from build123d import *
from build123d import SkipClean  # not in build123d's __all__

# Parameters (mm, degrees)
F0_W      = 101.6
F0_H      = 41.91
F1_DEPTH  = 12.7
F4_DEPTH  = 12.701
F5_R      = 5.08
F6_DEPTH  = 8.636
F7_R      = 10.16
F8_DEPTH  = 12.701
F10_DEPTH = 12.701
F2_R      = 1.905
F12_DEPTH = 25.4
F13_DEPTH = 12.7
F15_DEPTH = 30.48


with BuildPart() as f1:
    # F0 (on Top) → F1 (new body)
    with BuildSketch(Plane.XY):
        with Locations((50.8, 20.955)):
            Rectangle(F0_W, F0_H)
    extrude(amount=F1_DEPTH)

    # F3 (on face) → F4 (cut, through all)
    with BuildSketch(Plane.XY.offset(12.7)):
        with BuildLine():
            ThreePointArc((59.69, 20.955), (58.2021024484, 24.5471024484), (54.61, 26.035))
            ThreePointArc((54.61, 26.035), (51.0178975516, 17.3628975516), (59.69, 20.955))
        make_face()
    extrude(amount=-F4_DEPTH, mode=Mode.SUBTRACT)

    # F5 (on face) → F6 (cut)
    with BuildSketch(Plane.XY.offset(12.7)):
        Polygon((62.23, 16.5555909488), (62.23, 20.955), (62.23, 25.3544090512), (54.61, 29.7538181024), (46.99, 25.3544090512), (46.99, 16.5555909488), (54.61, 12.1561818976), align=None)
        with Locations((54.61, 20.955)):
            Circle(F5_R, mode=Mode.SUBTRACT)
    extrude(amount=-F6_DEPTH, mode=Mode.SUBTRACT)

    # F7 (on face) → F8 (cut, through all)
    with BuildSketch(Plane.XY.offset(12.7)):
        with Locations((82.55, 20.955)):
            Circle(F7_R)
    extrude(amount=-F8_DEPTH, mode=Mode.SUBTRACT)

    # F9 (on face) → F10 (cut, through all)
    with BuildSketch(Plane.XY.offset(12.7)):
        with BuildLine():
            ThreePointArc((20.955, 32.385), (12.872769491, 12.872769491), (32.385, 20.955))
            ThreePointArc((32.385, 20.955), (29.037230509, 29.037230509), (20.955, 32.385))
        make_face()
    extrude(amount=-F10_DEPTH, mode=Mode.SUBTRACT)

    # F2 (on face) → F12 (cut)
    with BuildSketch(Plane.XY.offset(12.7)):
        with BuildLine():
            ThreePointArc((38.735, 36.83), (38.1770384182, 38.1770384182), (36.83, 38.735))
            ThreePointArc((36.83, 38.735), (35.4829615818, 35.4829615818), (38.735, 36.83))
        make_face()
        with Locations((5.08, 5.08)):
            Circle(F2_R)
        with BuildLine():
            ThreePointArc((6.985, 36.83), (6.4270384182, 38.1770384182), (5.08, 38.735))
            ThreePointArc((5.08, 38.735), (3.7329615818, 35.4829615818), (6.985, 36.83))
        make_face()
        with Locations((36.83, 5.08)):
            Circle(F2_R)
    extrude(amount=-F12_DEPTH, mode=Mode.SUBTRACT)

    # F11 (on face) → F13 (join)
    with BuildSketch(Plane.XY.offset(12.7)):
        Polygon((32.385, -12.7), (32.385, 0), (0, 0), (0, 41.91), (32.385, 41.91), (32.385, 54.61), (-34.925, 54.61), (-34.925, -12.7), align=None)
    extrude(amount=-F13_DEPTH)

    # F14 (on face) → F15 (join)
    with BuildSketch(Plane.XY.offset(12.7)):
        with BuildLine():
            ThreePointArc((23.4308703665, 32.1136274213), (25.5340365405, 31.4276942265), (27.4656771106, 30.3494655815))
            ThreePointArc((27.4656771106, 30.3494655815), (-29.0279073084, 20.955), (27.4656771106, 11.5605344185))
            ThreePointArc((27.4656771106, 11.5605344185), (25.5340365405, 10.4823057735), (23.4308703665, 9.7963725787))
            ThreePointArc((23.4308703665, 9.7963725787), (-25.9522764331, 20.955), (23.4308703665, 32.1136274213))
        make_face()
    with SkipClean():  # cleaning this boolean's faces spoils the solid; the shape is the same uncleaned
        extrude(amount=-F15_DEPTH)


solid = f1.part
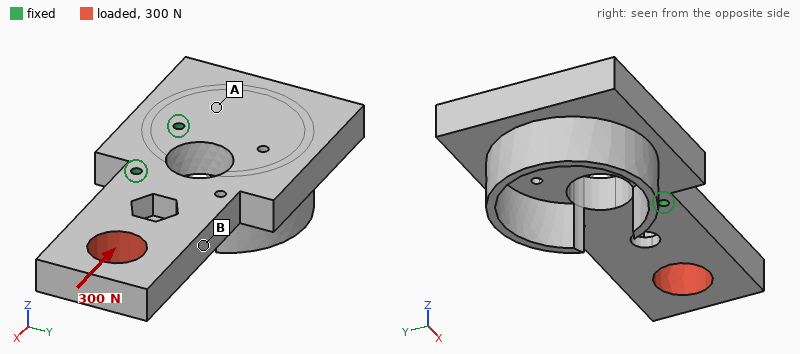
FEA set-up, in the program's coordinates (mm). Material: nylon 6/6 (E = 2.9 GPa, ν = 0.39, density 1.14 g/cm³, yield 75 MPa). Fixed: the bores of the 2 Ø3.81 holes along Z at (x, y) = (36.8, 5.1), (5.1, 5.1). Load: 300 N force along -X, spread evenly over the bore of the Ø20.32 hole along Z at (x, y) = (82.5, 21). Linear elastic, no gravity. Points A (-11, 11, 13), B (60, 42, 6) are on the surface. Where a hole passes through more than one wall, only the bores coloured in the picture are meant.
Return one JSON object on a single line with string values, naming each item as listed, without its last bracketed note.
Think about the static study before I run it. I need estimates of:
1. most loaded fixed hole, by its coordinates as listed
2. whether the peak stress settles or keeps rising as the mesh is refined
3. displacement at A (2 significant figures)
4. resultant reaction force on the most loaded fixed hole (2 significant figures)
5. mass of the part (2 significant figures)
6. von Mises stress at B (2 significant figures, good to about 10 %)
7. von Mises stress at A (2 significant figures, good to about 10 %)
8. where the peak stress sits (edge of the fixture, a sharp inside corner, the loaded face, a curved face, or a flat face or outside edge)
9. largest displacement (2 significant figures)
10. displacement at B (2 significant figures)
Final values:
{"most loaded fixed hole, by its coordinates as listed": "(36.8, 5.1)", "whether the peak stress settles or keeps rising as the mesh is refined": "keeps rising", "displacement at A": "14 µm", "resultant reaction force on the most loaded fixed hole": "220 N", "mass of the part": "100 g", "von Mises stress at B": "0.79 MPa", "von Mises stress at A": "0.32 MPa", "where the peak stress sits": "edge of the fixture", "largest displacement": "86 µm", "displacement at B": "55 µm"}
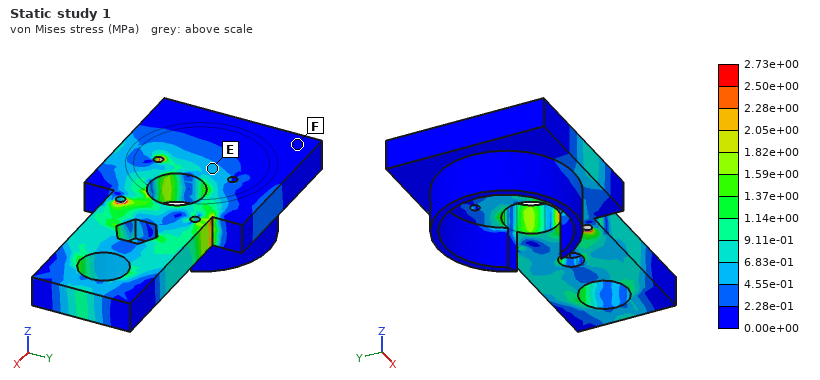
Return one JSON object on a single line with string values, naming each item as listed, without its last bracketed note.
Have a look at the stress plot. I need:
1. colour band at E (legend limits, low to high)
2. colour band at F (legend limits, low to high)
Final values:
{"colour band at E": "4.55e-01 to 6.83e-01 MPa", "colour band at F": "0.00e+00 to 2.28e-01 MPa"}
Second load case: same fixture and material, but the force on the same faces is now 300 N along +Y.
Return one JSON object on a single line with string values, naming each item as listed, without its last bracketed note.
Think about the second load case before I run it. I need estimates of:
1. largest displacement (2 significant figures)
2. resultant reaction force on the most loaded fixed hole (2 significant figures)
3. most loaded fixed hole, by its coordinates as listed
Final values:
{"largest displacement": "0.39 mm", "resultant reaction force on the most loaded fixed hole": "720 N", "most loaded fixed hole, by its coordinates as listed": "(36.8, 5.1)"}
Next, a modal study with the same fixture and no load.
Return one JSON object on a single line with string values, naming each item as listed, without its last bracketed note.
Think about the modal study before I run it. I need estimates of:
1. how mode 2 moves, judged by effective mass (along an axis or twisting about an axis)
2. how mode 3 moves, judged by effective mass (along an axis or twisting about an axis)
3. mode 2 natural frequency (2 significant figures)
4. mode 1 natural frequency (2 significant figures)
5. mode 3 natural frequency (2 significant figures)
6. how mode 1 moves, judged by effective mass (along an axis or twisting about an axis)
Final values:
{"how mode 2 moves, judged by effective mass": "along Z", "how mode 3 moves, judged by effective mass": "along X", "mode 2 natural frequency": "770 Hz", "mode 1 natural frequency": "580 Hz", "mode 3 natural frequency": "960 Hz", "how mode 1 moves, judged by effective mass": "along Z"}
